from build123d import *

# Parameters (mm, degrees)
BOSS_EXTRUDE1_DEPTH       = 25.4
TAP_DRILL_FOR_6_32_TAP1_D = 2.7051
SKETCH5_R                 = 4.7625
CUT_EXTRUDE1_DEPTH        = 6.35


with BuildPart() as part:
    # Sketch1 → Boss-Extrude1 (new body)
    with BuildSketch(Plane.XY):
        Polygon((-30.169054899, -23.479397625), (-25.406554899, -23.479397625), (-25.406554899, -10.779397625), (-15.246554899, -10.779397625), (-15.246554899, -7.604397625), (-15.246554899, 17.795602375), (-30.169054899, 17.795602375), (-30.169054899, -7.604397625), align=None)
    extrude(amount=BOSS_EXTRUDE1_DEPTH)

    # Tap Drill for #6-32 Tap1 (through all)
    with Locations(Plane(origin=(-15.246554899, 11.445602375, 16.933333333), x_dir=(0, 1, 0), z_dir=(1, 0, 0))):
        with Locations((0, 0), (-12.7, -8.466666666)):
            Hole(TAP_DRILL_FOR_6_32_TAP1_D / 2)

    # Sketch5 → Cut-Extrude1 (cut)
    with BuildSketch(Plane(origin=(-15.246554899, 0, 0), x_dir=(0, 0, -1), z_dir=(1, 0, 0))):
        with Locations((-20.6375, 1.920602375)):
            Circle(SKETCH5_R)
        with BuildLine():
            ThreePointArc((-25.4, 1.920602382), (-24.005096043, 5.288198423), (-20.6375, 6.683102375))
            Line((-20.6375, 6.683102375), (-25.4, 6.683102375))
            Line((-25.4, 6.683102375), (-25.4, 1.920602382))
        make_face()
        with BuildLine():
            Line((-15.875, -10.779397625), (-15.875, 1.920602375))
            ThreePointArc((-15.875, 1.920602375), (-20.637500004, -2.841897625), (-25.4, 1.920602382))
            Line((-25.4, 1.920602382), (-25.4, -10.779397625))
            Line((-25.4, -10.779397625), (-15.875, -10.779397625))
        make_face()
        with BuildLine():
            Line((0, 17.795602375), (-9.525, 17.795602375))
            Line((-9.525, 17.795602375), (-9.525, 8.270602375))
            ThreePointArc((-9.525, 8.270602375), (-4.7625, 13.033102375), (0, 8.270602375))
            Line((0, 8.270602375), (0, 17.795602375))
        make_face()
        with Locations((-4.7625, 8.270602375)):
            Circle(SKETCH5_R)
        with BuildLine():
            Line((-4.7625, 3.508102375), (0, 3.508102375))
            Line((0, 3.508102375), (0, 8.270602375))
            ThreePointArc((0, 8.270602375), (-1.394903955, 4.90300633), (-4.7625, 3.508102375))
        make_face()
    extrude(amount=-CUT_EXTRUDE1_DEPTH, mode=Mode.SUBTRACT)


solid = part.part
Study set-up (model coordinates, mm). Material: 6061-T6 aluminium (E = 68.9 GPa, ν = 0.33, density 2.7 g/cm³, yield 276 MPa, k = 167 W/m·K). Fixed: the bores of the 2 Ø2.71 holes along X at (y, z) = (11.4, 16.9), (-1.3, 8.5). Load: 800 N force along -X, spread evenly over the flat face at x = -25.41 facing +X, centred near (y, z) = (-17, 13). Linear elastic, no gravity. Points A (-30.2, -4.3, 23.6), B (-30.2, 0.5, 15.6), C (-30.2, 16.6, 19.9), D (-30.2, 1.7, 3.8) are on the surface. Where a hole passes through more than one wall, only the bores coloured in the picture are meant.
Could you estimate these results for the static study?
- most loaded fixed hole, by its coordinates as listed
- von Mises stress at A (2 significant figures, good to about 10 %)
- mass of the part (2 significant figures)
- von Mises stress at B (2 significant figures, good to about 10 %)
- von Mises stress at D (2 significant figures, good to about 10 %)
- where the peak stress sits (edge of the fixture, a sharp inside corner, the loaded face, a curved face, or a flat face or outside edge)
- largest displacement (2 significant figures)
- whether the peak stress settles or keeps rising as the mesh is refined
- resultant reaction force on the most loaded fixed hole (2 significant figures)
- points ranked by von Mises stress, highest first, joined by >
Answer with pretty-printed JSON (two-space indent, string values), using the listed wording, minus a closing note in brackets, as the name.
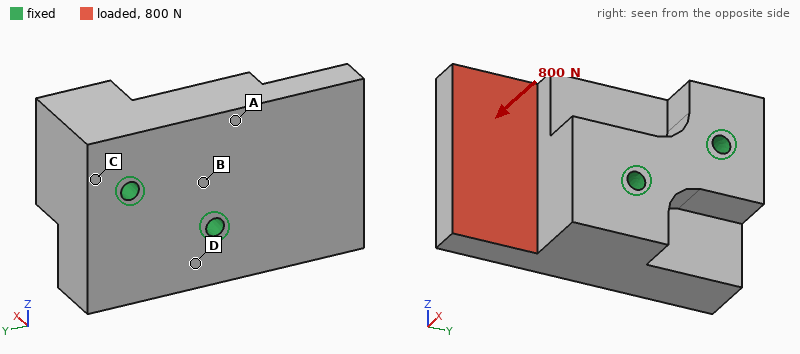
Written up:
{
  "most loaded fixed hole, by its coordinates as listed": "(-1.3, 8.5)",
  "von Mises stress at A": "18 MPa",
  "mass of the part": "28 g",
  "von Mises stress at B": "13 MPa",
  "von Mises stress at D": "7.9 MPa",
  "where the peak stress sits": "edge of the fixture",
  "largest displacement": "40 µm",
  "whether the peak stress settles or keeps rising as the mesh is refined": "keeps rising",
  "resultant reaction force on the most loaded fixed hole": "930 N",
  "points ranked by von Mises stress, highest first, joined by >": "A > B > D > C"
}
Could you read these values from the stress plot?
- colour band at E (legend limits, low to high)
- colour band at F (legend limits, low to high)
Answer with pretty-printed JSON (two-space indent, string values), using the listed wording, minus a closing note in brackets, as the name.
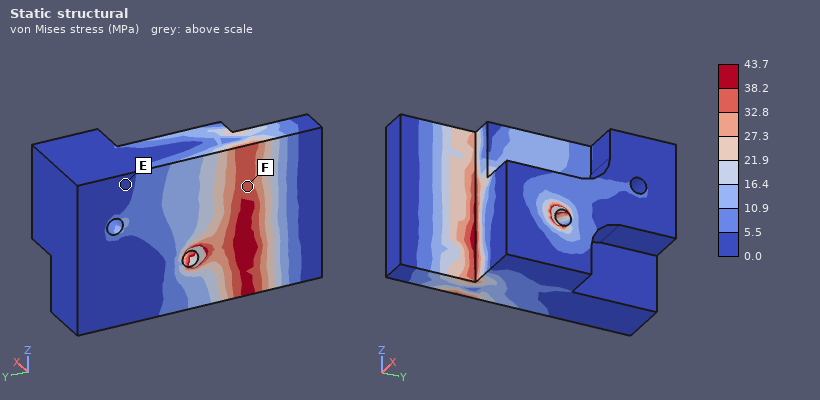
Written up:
{
  "colour band at E": "0.0 to 5.5 MPa",
  "colour band at F": "32.8 to 38.2 MPa"
}
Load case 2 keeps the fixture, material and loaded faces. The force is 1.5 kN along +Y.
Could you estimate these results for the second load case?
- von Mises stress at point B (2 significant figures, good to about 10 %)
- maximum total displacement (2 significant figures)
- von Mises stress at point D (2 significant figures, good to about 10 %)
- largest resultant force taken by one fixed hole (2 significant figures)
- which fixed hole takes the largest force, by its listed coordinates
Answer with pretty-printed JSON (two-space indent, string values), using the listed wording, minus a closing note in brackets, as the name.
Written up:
{
  "von Mises stress at point B": "5.6 MPa",
  "maximum total displacement": "18 µm",
  "von Mises stress at point D": "3.7 MPa",
  "largest resultant force taken by one fixed hole": "950 N",
  "which fixed hole takes the largest force, by its listed coordinates": "(-1.3, 8.5)"
}
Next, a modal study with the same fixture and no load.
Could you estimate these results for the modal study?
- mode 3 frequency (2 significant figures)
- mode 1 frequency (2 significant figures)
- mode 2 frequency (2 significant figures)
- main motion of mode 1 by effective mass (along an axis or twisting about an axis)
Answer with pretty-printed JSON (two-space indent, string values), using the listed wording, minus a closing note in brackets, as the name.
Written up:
{
  "mode 3 frequency": "21 kHz",
  "mode 1 frequency": "14 kHz",
  "mode 2 frequency": "21 kHz",
  "main motion of mode 1 by effective mass": "along X"
}
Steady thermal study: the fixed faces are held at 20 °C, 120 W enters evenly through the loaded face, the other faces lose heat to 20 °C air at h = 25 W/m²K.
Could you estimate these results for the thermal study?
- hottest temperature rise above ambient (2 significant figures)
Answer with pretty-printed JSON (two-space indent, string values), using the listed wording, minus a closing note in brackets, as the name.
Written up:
{
  "hottest temperature rise above ambient": "83 K"
}
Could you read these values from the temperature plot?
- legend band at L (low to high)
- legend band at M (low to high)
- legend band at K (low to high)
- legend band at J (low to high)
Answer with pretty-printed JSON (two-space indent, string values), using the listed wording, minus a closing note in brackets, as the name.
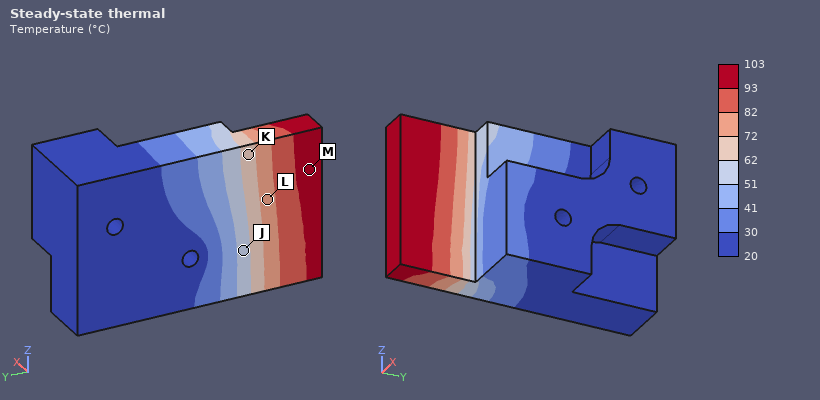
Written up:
{
  "legend band at L": "72 to 82 °C",
  "legend band at M": "93 to 103 °C",
  "legend band at K": "62 to 72 °C",
  "legend band at J": "51 to 62 °C"
}
